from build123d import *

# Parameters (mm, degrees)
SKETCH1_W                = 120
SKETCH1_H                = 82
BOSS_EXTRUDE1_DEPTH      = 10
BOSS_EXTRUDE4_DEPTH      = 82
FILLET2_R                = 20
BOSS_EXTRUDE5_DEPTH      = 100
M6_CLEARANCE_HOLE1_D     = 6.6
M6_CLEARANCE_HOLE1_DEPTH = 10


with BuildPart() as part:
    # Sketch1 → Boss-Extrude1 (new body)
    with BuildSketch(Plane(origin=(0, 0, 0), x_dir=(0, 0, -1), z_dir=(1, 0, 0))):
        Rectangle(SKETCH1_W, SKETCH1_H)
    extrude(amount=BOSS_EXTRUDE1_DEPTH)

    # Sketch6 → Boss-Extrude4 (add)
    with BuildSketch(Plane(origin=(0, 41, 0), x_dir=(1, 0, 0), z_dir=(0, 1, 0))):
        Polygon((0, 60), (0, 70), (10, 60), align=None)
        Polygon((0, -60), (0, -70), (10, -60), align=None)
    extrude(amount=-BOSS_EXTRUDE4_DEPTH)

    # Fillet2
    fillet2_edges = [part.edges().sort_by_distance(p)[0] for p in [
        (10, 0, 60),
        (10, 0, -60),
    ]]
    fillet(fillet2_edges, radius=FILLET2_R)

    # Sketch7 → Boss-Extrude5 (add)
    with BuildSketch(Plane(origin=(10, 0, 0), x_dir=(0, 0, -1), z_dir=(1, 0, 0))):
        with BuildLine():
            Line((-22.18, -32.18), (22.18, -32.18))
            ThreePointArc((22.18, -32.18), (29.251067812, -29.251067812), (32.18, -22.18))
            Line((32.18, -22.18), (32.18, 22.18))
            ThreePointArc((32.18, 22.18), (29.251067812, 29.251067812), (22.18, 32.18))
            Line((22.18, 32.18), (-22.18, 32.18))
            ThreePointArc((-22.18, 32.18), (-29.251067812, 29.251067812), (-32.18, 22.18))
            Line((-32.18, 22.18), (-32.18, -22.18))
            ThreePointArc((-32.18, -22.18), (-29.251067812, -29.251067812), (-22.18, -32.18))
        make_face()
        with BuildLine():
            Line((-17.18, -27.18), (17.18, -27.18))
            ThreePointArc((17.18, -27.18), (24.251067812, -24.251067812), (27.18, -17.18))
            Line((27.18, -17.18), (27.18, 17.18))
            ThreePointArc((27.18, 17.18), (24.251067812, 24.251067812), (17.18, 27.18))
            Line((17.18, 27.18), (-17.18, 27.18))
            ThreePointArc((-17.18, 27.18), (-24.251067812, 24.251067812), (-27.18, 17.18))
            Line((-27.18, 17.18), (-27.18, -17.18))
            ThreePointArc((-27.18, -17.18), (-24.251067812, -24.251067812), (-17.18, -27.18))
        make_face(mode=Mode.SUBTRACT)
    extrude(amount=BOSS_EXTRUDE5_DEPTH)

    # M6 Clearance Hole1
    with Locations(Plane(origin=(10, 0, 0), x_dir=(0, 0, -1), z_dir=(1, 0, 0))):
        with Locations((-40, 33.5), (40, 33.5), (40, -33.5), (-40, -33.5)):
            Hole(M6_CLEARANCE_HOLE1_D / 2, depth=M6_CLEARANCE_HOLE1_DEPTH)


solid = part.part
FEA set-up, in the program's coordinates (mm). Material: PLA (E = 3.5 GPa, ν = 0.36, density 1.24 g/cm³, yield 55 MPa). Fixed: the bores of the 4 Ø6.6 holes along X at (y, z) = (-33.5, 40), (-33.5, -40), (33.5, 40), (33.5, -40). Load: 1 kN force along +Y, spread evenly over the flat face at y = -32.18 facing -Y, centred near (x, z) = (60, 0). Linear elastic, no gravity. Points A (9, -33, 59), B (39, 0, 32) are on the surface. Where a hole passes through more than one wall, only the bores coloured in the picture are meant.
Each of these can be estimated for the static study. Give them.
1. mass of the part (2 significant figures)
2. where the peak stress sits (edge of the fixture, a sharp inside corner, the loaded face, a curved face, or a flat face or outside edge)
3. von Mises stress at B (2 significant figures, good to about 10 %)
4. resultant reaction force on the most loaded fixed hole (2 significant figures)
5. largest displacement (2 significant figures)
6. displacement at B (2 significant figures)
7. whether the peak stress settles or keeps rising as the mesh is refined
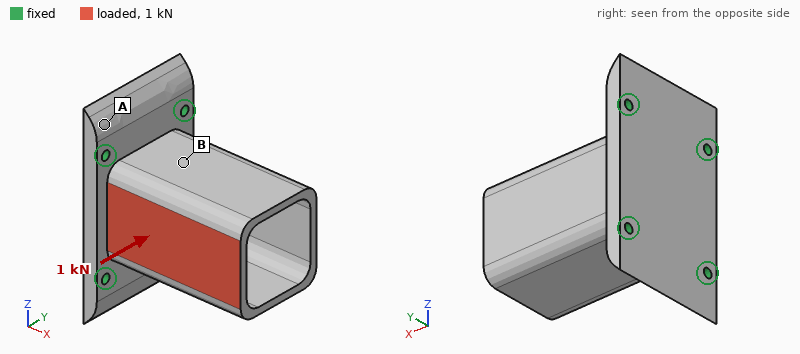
280 g
edge of the fixture
3.3 MPa
530 N
0.69 mm
0.13 mm
keeps rising
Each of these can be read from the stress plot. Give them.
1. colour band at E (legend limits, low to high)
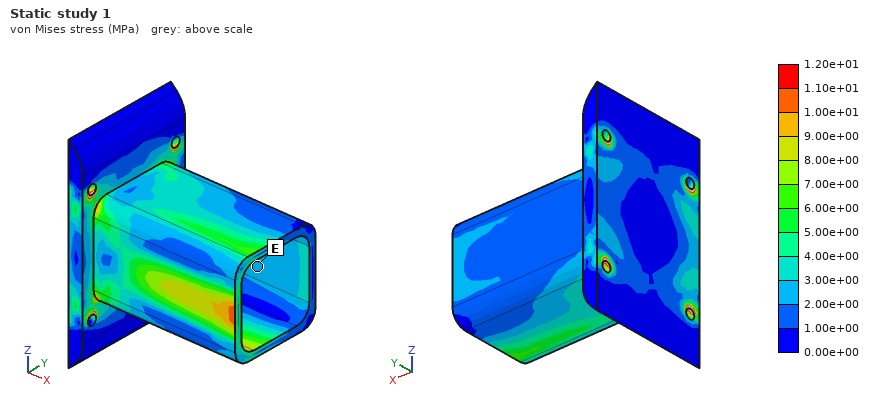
2.00e+00 to 3.00e+00 MPa
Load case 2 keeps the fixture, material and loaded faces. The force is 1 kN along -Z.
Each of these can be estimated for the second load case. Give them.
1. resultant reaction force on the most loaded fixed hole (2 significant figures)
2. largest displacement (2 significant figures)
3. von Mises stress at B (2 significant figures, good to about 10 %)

670 N
0.39 mm
1.6 MPa
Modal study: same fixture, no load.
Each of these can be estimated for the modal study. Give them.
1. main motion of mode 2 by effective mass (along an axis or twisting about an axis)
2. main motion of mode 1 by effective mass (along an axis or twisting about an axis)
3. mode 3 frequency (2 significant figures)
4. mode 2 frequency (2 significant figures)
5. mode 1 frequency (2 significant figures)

along Z
along Y
1200 Hz
940 Hz
830 Hz
